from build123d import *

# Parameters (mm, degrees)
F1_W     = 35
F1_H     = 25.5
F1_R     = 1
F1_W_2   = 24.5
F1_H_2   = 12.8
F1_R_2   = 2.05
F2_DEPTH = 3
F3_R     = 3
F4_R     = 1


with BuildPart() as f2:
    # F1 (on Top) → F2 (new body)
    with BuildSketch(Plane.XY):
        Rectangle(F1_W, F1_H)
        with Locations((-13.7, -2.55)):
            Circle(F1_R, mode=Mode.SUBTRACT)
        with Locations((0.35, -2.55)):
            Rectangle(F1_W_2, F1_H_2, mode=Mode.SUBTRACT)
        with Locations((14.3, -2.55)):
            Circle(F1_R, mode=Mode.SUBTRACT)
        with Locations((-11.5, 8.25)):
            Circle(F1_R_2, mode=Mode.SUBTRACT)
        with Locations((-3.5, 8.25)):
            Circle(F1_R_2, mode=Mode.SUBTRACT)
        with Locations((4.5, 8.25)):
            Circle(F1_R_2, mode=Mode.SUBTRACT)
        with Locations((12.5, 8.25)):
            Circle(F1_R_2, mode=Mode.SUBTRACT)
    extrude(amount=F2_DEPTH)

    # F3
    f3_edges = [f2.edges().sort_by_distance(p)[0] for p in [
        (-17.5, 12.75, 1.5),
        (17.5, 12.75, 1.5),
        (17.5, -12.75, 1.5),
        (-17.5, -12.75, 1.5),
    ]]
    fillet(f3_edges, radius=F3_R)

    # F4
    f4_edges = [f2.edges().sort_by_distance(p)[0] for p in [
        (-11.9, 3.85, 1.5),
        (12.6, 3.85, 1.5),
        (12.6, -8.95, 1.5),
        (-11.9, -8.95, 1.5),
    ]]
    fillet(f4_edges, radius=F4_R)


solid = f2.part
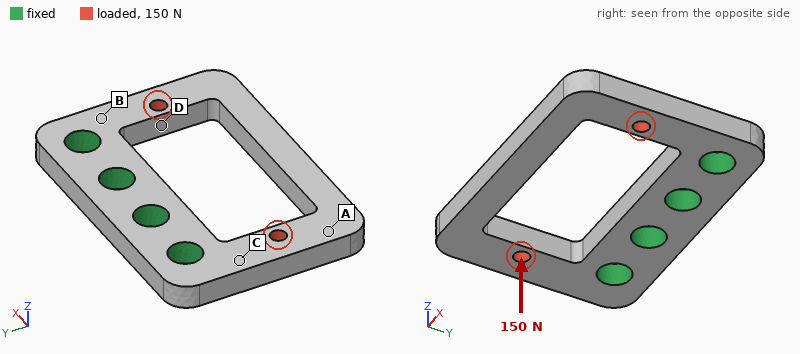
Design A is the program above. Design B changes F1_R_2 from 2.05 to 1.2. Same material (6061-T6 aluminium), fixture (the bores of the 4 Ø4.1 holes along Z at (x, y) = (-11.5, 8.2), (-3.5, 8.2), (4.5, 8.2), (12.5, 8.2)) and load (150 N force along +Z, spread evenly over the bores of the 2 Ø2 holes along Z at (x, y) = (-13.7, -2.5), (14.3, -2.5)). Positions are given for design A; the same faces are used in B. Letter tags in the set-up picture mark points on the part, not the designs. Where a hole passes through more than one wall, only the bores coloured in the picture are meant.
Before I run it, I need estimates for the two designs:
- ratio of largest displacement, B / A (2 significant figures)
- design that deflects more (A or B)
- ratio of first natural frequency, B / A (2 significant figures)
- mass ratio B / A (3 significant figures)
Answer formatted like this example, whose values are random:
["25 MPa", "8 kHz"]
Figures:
["1.2", "B", "0.94", "1.07"]
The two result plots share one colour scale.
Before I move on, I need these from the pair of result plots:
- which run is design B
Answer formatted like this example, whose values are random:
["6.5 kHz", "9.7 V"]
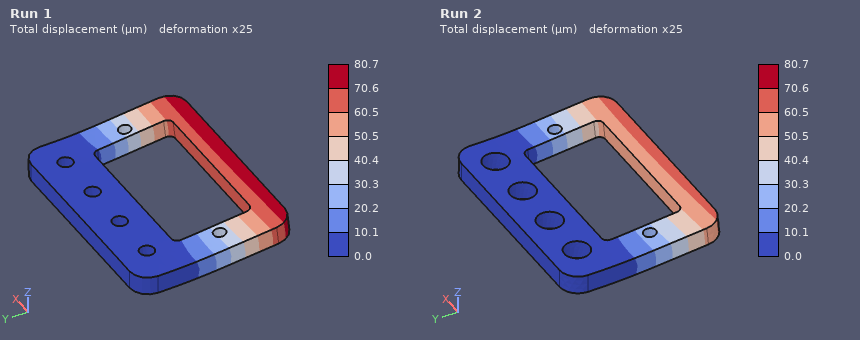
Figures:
["Run 1"]
